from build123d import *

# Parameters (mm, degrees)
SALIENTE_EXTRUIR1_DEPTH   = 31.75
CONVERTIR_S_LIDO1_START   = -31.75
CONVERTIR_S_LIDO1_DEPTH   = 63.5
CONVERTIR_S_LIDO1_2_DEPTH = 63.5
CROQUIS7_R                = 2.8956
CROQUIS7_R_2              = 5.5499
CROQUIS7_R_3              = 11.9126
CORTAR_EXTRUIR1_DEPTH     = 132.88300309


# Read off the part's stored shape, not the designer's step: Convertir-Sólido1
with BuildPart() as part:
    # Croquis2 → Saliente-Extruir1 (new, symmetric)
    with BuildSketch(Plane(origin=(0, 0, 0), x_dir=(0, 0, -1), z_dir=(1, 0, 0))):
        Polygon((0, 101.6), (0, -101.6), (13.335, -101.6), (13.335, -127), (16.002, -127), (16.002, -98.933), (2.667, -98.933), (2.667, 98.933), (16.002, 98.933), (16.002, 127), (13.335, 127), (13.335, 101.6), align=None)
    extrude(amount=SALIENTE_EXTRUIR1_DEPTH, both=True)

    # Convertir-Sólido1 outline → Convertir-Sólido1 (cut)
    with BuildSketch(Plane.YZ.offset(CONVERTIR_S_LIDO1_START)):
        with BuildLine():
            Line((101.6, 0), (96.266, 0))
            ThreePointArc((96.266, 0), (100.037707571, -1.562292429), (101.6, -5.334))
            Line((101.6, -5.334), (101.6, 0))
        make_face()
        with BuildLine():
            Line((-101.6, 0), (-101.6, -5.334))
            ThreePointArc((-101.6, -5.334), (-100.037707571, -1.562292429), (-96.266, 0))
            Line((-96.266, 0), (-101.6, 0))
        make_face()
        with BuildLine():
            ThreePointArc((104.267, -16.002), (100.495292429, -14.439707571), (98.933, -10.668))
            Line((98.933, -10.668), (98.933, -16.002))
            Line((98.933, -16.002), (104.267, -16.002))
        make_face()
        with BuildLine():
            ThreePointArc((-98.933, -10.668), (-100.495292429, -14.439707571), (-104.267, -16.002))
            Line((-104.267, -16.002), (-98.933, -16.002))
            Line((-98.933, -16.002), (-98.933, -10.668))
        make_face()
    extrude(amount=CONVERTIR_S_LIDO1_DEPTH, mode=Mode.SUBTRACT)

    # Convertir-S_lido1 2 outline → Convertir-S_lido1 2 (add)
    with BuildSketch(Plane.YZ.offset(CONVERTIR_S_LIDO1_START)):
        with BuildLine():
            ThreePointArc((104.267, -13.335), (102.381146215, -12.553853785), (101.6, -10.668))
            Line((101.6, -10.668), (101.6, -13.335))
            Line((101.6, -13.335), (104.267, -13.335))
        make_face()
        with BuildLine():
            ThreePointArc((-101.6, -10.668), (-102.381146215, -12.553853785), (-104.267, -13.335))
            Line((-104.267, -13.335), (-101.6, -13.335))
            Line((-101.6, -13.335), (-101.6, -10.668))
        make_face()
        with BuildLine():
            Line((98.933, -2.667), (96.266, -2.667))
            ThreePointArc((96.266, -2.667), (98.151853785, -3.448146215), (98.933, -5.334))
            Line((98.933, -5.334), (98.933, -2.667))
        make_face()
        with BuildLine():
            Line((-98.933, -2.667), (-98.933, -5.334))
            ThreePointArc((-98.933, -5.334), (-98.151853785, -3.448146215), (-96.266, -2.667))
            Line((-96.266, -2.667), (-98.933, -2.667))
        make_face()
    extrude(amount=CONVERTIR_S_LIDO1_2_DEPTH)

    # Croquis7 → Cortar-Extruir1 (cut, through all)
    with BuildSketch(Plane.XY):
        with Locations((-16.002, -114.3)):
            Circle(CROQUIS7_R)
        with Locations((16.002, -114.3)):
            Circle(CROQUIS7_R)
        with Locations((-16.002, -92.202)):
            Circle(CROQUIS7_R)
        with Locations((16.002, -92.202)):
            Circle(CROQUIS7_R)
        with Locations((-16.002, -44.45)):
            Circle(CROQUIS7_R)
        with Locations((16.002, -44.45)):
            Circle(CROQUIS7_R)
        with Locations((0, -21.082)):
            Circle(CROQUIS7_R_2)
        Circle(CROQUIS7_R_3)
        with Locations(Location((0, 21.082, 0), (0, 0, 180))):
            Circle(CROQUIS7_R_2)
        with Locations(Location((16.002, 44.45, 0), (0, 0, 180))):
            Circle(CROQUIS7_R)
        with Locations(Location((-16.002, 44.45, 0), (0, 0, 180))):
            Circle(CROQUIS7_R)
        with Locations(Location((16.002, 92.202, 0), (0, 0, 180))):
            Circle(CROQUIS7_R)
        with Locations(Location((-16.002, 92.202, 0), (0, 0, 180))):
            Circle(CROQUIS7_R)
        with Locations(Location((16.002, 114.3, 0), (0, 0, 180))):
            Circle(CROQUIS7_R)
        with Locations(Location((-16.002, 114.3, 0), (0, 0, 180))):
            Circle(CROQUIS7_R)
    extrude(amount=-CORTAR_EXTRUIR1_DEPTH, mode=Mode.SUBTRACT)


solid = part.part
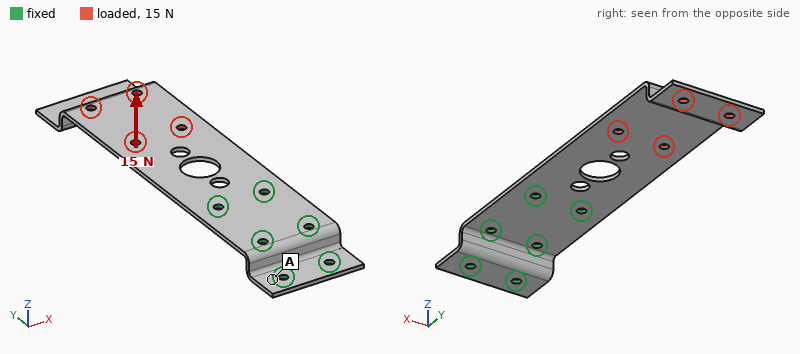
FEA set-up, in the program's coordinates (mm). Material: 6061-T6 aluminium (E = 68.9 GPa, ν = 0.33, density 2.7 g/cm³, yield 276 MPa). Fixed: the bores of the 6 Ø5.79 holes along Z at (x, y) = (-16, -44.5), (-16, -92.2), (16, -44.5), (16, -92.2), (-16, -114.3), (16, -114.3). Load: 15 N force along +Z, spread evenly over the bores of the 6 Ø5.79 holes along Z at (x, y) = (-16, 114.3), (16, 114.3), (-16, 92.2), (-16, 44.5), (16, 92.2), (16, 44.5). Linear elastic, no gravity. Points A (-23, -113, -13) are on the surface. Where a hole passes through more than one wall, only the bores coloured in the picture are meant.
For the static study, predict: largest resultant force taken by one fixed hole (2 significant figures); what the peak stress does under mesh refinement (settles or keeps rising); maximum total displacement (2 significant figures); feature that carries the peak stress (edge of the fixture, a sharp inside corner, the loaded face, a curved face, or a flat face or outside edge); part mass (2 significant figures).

9.5 N
keeps rising
2.7 mm
edge of the fixture
120 g
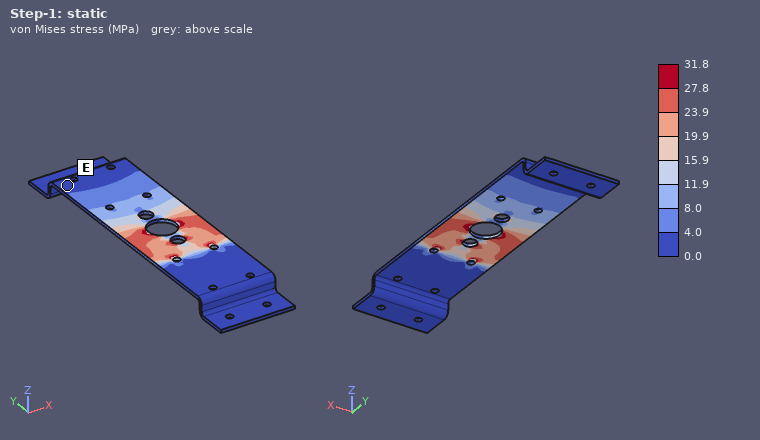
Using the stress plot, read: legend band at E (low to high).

0.0 to 4.0 MPa
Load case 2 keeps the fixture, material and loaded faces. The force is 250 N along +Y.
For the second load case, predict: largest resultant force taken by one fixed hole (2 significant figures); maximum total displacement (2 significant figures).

110 N
2.7 mm
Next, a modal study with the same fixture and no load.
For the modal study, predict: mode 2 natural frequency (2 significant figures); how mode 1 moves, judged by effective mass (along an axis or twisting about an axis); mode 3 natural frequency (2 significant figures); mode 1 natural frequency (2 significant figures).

340 Hz
along Z
450 Hz
65 Hz
